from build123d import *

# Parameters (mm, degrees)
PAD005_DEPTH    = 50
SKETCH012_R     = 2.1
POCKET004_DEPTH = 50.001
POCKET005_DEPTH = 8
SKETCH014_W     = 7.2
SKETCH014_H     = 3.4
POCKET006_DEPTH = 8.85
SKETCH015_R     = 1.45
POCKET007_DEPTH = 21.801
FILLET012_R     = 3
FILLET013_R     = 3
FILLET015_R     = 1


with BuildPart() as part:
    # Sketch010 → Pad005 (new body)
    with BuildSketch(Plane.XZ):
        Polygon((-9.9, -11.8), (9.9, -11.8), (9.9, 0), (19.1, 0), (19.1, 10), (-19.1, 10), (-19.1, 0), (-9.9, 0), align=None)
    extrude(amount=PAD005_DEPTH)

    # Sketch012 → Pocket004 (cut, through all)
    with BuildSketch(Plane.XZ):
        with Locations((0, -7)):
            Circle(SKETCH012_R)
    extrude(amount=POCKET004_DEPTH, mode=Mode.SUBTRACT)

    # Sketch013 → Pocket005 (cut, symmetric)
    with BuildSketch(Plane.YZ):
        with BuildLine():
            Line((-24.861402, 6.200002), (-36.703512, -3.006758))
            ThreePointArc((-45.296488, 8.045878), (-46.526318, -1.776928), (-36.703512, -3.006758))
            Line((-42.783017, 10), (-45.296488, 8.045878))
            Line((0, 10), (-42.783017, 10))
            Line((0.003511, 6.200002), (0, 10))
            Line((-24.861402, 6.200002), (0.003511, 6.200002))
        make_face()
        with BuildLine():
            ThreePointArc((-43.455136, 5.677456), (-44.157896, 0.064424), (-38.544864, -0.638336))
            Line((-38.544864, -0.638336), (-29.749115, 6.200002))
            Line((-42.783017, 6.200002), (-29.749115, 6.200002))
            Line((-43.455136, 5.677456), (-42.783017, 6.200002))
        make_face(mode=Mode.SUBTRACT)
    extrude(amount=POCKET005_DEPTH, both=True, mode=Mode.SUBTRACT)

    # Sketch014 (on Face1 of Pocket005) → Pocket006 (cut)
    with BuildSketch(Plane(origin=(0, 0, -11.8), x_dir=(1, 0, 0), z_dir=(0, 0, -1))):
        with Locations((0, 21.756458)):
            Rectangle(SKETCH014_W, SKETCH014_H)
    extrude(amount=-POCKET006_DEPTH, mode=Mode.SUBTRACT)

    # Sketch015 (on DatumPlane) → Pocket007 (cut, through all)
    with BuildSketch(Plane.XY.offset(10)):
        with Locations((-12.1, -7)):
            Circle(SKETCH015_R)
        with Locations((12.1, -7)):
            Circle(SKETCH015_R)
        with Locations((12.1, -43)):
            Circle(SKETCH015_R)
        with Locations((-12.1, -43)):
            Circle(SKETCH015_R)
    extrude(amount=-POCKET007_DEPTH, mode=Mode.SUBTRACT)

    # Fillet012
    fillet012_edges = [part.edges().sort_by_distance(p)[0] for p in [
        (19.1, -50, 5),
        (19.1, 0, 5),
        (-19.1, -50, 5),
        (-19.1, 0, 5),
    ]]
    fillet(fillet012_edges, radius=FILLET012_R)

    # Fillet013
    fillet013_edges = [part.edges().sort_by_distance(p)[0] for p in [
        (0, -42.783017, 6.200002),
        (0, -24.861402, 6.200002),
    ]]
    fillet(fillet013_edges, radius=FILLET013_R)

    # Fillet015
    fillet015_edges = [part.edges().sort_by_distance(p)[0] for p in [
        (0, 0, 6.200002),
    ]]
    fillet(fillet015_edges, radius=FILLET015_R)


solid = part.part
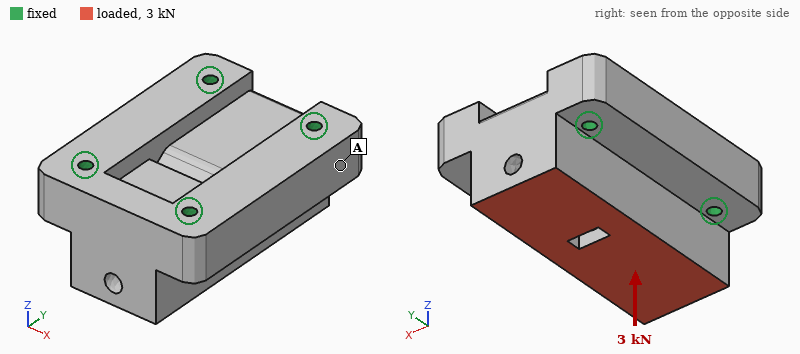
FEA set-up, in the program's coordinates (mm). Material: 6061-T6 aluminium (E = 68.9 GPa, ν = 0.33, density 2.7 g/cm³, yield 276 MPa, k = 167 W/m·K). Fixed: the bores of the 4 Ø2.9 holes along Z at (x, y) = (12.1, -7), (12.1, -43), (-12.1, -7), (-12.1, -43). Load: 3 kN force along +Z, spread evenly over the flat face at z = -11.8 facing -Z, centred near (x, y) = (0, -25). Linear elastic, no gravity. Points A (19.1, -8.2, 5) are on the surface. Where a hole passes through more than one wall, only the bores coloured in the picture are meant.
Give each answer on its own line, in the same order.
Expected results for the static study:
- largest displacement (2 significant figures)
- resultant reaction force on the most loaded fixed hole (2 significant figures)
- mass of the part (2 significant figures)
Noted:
3.8 µm
820 N
69 g
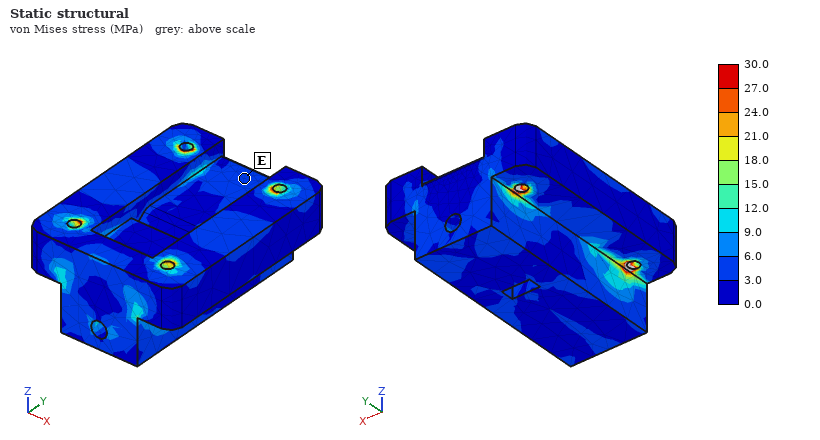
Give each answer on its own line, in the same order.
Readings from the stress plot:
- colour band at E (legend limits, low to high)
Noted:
3.0 to 6.0 MPa
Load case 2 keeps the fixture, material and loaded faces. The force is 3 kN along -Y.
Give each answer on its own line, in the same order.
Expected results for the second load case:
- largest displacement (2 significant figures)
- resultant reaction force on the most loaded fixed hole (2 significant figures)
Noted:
7.6 µm
1.1 kN
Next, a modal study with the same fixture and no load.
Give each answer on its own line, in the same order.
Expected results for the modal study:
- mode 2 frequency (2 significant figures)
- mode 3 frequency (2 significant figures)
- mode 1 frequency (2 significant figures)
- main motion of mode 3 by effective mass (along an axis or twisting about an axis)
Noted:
23 kHz
26 kHz
23 kHz
along Y
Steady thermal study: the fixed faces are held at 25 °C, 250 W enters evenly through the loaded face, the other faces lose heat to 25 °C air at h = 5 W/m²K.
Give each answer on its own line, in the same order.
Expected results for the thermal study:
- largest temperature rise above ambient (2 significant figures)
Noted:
54 K
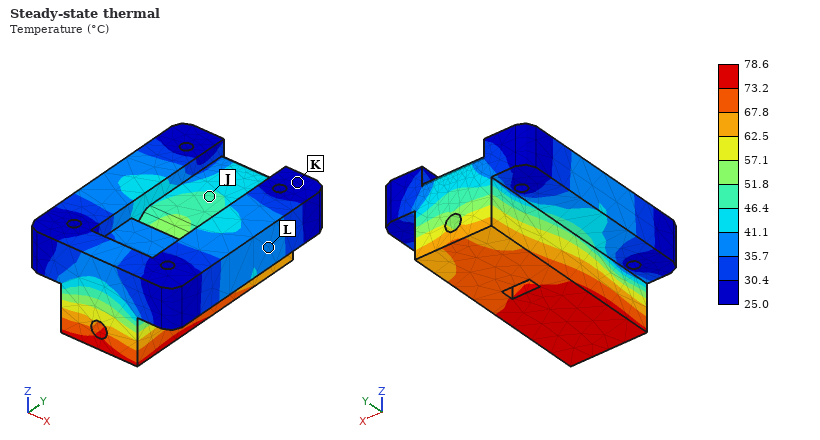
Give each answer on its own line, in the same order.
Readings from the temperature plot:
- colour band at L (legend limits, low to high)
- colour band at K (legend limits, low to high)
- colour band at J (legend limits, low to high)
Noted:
35.7 to 41.1 °C
25.0 to 30.4 °C
46.4 to 51.8 °C
